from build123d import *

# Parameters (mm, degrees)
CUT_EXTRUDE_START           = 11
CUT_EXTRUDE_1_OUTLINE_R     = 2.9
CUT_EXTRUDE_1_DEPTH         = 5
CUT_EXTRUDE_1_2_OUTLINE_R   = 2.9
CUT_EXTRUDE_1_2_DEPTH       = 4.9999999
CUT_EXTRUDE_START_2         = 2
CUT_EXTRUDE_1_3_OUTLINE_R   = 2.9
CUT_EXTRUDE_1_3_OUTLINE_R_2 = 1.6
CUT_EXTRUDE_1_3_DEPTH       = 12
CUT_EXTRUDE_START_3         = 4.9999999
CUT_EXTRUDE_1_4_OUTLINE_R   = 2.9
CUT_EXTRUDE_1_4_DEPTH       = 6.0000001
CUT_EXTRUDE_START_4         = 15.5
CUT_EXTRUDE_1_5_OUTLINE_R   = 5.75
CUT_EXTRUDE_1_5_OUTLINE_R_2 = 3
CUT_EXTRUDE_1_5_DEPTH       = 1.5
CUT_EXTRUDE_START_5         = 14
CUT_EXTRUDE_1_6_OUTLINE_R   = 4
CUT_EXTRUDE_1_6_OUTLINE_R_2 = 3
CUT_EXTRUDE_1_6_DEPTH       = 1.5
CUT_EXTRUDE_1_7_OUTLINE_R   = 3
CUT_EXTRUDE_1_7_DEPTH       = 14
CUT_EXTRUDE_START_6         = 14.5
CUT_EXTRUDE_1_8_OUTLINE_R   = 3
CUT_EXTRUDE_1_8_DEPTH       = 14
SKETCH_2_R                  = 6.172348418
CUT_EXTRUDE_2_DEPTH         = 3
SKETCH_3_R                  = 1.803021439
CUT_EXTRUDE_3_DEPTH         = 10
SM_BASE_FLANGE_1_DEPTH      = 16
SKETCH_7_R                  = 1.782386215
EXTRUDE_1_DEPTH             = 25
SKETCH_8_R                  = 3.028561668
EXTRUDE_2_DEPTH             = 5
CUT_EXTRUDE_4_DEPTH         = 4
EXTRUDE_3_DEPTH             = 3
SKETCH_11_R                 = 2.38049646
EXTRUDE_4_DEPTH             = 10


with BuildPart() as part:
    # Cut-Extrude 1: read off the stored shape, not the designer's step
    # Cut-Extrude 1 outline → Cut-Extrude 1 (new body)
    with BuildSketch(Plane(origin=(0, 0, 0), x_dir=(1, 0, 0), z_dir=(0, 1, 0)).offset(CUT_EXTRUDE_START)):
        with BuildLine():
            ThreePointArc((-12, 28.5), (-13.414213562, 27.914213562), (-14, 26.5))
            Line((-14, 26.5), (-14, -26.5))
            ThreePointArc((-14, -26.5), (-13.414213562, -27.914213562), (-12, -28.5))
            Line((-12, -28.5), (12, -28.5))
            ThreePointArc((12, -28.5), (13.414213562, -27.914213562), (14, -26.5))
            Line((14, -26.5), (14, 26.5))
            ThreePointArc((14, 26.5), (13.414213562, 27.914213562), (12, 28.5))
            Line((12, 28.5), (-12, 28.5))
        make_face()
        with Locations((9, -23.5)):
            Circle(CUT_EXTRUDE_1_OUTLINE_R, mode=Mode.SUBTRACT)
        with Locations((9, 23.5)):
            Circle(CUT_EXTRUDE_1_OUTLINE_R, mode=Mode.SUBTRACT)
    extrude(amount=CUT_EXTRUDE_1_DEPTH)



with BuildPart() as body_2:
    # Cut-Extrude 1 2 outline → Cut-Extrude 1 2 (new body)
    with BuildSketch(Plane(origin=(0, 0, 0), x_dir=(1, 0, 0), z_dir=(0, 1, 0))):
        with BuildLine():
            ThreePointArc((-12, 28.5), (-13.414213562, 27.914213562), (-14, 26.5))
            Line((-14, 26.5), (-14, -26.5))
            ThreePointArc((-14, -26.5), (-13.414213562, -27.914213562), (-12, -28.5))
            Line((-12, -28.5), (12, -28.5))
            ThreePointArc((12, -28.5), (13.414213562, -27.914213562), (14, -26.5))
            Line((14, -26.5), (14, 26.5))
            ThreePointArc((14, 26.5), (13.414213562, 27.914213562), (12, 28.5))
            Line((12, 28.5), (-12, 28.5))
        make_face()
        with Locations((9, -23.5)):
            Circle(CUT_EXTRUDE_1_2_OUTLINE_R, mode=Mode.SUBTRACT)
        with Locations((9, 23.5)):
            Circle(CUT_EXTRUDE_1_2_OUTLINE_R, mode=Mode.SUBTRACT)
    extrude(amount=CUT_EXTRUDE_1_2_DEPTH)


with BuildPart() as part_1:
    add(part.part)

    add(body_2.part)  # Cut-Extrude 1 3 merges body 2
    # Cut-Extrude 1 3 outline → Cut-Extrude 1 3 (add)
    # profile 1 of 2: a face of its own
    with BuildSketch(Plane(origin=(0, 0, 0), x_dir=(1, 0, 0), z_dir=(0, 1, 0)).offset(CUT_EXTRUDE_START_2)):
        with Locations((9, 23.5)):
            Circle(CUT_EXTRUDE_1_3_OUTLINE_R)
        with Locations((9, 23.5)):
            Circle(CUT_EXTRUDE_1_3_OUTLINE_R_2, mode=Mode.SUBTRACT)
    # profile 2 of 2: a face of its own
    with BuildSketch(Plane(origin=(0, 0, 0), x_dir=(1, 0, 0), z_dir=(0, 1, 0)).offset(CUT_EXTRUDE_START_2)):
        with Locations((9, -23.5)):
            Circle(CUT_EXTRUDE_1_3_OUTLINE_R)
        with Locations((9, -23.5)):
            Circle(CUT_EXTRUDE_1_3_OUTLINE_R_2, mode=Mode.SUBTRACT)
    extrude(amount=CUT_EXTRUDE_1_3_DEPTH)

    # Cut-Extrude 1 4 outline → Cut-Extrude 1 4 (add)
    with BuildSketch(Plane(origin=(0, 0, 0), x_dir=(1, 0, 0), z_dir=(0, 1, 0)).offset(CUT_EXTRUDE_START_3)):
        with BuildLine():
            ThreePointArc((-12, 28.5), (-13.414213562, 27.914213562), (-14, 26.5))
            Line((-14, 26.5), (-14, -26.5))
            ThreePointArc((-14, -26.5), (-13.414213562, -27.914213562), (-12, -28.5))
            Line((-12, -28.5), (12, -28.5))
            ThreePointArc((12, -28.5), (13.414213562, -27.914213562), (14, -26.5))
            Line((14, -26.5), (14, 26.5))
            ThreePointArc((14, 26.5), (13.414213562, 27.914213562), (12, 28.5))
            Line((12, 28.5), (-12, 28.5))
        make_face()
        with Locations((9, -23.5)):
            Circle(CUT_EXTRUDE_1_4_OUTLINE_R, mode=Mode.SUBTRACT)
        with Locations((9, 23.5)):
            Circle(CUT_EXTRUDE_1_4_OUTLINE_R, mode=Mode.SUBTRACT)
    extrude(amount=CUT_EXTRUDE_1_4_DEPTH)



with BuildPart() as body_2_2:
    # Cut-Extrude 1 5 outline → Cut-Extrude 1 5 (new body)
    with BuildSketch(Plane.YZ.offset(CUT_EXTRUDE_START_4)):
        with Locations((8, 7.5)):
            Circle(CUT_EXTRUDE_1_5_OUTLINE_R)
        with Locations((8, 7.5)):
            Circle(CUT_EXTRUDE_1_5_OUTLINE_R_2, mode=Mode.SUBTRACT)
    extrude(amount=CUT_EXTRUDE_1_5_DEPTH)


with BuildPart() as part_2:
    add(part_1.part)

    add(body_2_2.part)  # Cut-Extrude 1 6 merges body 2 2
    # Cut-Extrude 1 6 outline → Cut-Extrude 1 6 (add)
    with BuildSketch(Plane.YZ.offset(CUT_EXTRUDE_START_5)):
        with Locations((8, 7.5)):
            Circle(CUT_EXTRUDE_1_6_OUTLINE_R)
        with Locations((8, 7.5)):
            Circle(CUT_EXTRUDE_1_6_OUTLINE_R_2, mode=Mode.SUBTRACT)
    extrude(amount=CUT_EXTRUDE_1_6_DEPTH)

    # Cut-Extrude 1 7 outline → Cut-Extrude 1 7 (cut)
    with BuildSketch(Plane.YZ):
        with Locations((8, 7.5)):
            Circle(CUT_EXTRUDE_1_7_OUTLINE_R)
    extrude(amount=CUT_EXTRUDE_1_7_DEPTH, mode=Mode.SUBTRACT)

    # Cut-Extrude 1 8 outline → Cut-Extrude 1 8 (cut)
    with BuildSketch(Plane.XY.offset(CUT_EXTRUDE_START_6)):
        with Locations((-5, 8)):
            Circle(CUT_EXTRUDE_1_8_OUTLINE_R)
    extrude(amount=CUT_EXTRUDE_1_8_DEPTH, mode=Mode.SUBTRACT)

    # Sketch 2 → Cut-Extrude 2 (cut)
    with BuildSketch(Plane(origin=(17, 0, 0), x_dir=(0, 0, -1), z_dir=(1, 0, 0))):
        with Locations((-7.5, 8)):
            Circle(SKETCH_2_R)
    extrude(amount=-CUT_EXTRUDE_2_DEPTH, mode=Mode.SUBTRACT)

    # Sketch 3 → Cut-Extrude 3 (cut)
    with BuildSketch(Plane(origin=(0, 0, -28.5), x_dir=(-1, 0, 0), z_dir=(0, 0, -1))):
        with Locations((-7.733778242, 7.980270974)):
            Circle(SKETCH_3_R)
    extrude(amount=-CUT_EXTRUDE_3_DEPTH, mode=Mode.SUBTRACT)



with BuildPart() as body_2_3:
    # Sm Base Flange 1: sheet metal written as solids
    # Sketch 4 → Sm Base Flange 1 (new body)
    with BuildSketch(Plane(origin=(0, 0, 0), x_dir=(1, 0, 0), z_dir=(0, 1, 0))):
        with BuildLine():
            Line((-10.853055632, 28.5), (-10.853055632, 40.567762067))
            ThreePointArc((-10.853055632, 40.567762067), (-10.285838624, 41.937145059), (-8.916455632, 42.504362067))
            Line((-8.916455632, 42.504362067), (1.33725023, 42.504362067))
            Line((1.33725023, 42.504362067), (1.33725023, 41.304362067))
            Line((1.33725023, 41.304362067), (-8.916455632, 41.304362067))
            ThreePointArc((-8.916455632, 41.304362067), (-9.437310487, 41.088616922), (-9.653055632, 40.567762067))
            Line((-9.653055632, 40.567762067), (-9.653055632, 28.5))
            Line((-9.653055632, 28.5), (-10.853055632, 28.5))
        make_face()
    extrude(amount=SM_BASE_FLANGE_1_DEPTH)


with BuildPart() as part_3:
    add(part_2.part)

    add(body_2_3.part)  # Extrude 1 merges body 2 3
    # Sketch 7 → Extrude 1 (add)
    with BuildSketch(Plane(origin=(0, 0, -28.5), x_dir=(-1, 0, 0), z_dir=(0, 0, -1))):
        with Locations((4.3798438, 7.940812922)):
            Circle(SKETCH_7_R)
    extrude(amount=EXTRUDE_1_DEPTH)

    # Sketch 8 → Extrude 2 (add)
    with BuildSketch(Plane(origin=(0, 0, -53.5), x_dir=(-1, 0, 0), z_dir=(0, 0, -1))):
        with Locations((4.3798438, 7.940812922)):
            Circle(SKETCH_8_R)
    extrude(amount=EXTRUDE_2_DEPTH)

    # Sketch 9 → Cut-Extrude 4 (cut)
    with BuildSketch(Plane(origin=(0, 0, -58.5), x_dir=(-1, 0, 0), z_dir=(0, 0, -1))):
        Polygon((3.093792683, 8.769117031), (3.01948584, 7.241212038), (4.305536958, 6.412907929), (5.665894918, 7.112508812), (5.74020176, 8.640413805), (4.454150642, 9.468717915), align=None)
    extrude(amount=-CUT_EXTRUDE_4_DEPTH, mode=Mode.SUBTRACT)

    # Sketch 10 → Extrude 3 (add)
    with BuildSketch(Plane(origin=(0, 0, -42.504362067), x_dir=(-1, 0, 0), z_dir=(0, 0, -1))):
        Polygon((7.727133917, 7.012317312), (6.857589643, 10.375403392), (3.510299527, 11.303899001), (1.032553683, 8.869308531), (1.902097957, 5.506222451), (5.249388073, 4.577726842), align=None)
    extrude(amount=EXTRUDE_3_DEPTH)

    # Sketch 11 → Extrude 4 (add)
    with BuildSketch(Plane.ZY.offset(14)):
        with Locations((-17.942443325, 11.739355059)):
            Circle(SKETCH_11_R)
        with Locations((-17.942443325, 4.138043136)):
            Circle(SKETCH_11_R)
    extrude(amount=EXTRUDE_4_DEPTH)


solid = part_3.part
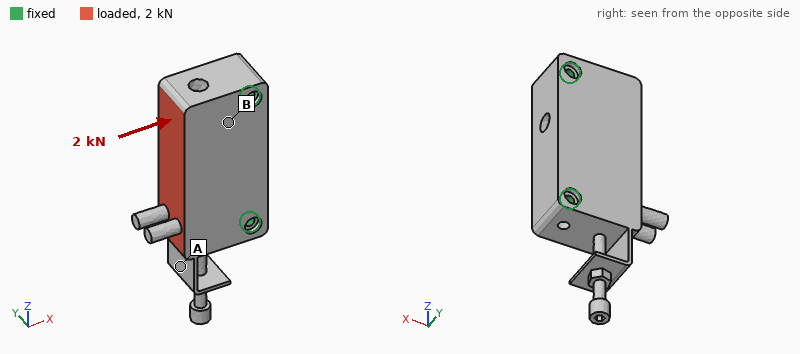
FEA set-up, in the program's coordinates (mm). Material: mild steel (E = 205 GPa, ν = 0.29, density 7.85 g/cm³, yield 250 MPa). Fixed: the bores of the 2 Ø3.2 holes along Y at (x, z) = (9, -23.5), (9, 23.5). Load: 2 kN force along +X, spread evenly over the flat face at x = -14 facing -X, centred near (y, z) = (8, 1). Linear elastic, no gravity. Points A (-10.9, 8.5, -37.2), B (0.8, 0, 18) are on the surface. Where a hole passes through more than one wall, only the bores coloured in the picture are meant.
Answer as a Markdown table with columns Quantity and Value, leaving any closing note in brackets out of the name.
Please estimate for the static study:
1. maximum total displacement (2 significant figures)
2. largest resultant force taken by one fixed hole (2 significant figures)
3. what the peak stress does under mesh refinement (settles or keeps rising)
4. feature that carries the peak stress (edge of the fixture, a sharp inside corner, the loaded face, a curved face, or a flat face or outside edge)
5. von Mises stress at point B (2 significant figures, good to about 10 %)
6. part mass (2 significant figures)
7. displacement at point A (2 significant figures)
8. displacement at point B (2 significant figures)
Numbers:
| Quantity | Value |
|---|---|
| maximum total displacement | 0.88 µm |
| largest resultant force taken by one fixed hole | 1.1 kN |
| what the peak stress does under mesh refinement | keeps rising |
| feature that carries the peak stress | edge of the fixture |
| von Mises stress at point B | 4.6 MPa |
| part mass | 200 g |
| displacement at point A | 0.19 µm |
| displacement at point B | 0.44 µm |
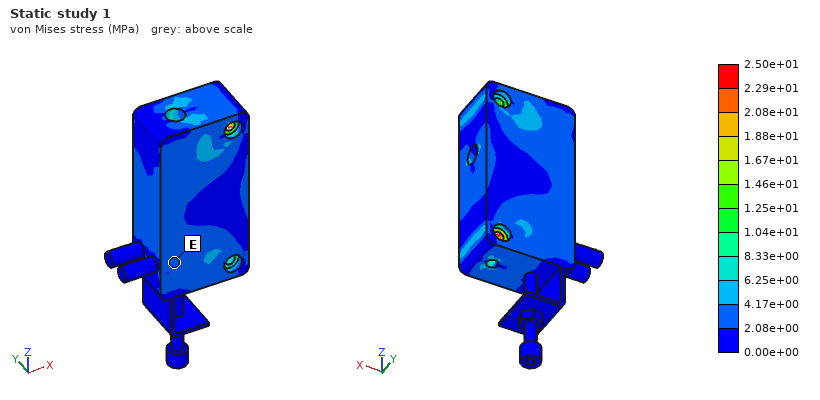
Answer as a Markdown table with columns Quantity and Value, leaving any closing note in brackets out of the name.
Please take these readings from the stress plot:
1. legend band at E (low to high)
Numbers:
| Quantity | Value |
|---|---|
| legend band at E | 2.08e+00 to 4.17e+00 MPa |
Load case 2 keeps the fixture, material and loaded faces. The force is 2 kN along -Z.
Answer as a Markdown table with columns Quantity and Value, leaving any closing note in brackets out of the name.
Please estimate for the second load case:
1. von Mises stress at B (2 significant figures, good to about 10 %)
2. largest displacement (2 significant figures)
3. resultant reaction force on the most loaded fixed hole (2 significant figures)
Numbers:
| Quantity | Value |
|---|---|
| von Mises stress at B | 4.7 MPa |
| largest displacement | 2.4 µm |
| resultant reaction force on the most loaded fixed hole | 1.4 kN |
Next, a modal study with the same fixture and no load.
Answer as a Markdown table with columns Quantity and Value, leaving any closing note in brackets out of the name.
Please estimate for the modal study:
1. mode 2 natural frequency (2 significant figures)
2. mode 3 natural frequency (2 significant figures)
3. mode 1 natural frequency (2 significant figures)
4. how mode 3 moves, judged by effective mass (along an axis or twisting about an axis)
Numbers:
| Quantity | Value |
|---|---|
| mode 2 natural frequency | 4300 Hz |
| mode 3 natural frequency | 8800 Hz |
| mode 1 natural frequency | 4300 Hz |
| how mode 3 moves, judged by effective mass | along Y |
